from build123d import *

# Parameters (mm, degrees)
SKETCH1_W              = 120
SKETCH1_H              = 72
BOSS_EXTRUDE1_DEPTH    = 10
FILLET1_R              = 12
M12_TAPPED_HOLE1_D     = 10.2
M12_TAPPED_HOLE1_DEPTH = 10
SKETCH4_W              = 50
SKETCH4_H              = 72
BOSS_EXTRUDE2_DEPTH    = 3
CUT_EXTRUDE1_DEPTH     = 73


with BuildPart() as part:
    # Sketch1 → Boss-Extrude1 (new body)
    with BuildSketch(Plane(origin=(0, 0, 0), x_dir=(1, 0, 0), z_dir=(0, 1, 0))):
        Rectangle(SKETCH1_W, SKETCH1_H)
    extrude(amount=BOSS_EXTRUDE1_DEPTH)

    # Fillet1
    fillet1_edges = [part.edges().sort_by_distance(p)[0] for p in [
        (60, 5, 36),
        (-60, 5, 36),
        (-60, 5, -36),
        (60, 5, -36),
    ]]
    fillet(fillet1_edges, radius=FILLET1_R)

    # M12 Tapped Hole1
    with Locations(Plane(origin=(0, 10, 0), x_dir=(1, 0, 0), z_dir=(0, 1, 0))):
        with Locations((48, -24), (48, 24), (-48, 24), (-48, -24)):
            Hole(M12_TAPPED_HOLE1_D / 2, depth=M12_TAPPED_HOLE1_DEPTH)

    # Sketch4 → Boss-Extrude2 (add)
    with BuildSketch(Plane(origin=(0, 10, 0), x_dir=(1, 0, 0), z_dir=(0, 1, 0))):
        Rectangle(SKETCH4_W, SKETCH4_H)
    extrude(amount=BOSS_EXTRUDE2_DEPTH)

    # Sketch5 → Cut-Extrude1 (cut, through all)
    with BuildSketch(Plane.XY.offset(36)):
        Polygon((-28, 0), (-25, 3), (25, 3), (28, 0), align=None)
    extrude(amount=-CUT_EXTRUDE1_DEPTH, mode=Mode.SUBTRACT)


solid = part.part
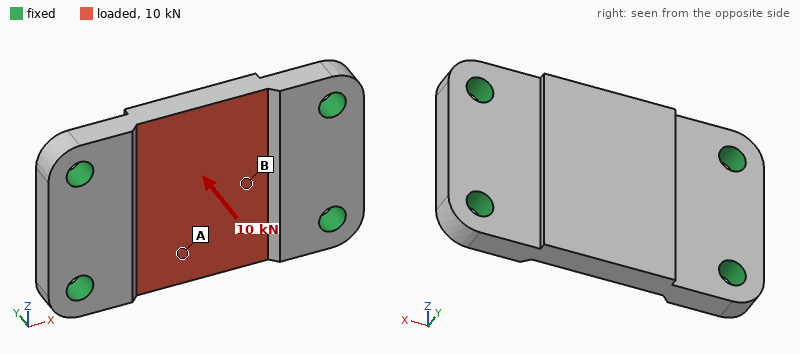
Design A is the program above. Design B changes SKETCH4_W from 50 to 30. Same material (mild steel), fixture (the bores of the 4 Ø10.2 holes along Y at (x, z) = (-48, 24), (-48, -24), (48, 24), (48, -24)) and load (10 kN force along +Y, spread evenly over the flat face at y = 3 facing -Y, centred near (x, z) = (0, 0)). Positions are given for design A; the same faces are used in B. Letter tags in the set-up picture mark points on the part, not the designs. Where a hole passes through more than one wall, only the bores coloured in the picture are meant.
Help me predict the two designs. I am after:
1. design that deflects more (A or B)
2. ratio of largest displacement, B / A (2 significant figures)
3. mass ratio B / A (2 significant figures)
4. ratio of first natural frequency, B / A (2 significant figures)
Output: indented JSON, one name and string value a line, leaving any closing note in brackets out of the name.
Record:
{
  "design that deflects more": "B",
  "ratio of largest displacement, B / A": "1.1",
  "mass ratio B / A": "0.95",
  "ratio of first natural frequency, B / A": "0.97"
}
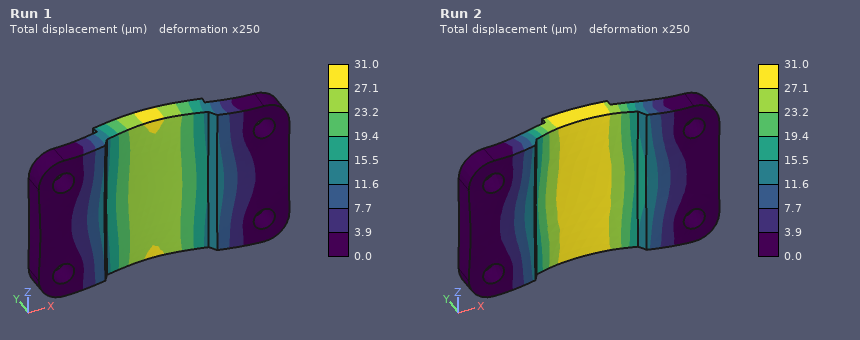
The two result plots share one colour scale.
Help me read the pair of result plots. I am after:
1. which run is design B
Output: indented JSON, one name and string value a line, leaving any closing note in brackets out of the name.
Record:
{
  "which run is design B": "Run 2"
}
